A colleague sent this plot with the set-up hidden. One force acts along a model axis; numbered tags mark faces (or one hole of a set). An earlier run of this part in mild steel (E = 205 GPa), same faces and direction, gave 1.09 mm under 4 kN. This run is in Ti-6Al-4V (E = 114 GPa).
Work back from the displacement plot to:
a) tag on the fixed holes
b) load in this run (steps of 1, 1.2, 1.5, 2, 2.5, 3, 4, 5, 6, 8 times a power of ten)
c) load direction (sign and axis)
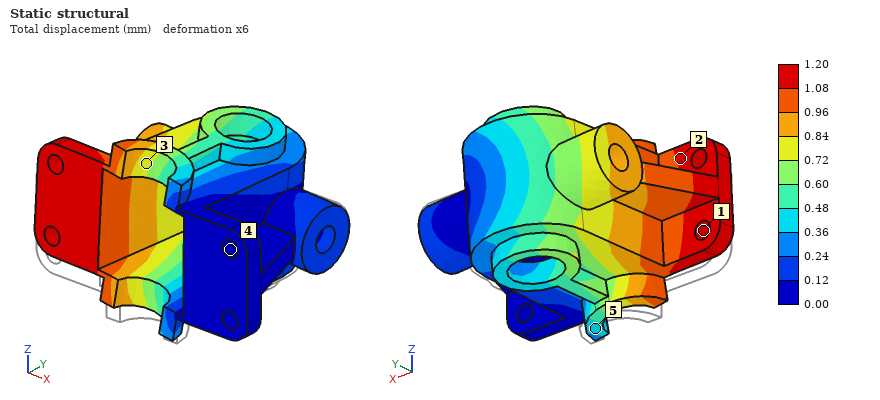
4
2.5 kN
+Z
